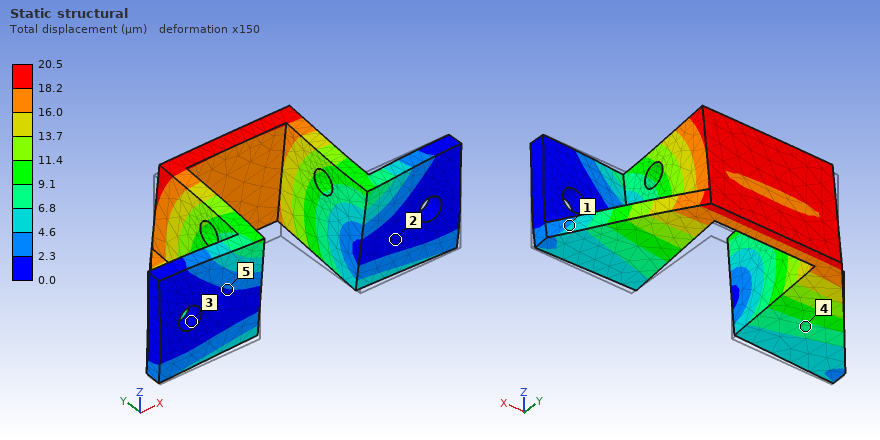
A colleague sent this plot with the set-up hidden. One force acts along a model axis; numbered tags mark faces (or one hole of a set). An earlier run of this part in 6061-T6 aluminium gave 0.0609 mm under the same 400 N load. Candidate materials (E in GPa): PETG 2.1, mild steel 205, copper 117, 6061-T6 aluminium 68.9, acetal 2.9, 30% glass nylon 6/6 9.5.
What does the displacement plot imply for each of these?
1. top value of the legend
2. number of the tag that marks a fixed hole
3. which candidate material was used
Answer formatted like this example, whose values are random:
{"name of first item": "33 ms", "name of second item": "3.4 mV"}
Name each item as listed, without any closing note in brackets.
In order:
{"top value of the legend": "20.5 µm", "number of the tag that marks a fixed hole": "3", "which candidate material was used": "mild steel"}
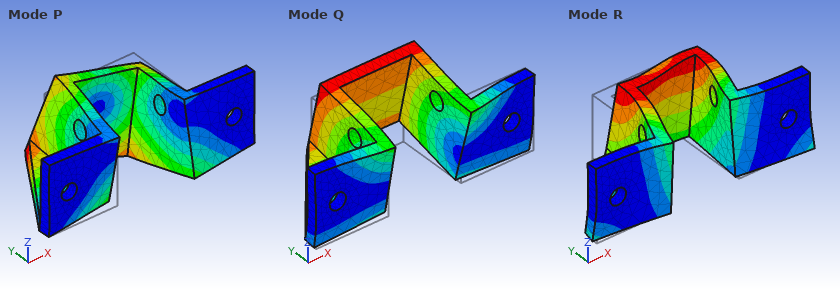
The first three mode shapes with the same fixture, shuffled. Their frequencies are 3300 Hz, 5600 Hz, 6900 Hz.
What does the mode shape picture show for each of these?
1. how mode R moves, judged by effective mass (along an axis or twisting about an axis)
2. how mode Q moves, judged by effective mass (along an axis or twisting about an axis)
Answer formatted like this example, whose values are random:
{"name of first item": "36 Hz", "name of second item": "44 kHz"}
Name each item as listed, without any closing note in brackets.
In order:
{"how mode R moves, judged by effective mass": "along X", "how mode Q moves, judged by effective mass": "along Z"}
